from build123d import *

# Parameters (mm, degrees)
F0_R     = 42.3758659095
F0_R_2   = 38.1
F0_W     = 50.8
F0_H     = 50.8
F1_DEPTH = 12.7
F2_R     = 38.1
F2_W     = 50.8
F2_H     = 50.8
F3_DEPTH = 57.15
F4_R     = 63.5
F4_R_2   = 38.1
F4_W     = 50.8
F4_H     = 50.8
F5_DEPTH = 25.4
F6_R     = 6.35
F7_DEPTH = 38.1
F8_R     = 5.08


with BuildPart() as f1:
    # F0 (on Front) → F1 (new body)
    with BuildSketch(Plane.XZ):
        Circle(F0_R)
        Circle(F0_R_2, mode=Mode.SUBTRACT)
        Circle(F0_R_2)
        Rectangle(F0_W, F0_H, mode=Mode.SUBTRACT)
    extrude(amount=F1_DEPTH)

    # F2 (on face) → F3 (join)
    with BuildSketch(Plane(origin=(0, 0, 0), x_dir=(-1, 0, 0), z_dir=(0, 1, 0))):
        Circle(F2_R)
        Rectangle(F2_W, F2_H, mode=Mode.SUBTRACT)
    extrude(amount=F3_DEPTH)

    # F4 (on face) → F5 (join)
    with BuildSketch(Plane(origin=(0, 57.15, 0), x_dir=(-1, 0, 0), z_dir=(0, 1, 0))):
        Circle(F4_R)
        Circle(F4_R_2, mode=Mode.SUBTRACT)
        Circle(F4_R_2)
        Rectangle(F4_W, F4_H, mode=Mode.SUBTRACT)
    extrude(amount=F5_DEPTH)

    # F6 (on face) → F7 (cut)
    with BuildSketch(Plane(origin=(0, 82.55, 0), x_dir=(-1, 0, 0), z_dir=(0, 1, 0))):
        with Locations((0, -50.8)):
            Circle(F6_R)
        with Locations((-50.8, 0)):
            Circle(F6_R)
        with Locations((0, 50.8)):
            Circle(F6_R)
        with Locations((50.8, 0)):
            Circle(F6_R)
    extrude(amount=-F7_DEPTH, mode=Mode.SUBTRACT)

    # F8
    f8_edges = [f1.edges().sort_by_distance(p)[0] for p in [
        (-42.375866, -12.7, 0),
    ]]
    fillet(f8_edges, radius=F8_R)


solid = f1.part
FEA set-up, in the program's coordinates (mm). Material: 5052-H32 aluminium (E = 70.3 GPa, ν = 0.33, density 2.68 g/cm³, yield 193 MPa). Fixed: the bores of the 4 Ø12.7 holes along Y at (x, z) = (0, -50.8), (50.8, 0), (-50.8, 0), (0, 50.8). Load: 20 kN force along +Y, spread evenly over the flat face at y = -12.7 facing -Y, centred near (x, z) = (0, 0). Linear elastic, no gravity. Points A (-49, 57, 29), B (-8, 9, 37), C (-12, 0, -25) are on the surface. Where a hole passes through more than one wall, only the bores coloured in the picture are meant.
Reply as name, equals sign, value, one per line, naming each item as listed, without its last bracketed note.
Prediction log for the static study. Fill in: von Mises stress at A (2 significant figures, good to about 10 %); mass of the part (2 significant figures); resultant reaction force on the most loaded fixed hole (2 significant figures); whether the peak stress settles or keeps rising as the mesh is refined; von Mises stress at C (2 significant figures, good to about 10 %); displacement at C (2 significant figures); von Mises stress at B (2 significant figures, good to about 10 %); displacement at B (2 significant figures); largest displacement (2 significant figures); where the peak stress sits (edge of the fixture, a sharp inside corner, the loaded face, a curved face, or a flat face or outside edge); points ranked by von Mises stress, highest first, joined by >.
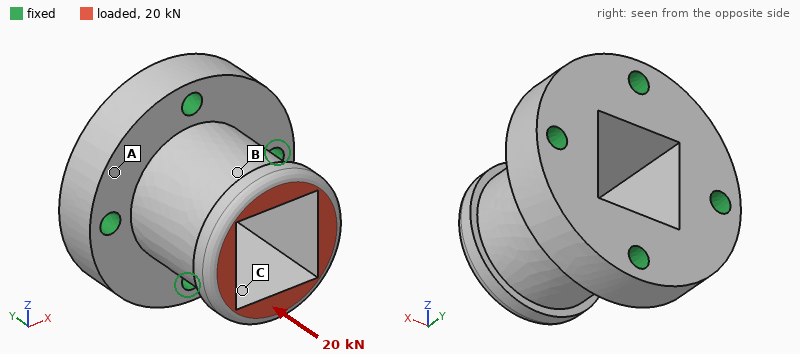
von Mises stress at A = 2.6 MPa
mass of the part = 1.1 kg
resultant reaction force on the most loaded fixed hole = 5.1 kN
whether the peak stress settles or keeps rising as the mesh is refined = keeps rising
von Mises stress at C = 12 MPa
displacement at C = 13 µm
von Mises stress at B = 8.4 MPa
displacement at B = 12 µm
largest displacement = 16 µm
where the peak stress sits = edge of the fixture
points ranked by von Mises stress, highest first, joined by > = C > B > A
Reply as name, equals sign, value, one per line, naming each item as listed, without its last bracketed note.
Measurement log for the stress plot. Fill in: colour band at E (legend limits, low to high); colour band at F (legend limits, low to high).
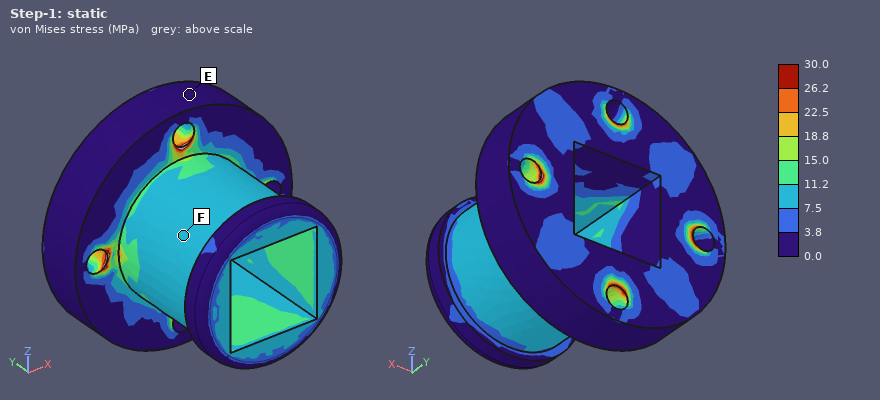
colour band at E = 0.0 to 3.8 MPa
colour band at F = 7.5 to 11.2 MPa
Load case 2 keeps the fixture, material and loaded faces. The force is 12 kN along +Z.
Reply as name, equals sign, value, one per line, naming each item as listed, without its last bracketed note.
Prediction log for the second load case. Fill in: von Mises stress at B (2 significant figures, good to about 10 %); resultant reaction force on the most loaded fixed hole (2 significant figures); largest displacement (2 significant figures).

von Mises stress at B = 19 MPa
resultant reaction force on the most loaded fixed hole = 10 kN
largest displacement = 0.10 mm
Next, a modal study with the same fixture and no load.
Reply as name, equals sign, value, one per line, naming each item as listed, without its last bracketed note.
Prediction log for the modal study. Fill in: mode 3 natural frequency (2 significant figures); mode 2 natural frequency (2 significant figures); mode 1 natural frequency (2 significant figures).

mode 3 natural frequency = 4900 Hz
mode 2 natural frequency = 4800 Hz
mode 1 natural frequency = 4800 Hz
